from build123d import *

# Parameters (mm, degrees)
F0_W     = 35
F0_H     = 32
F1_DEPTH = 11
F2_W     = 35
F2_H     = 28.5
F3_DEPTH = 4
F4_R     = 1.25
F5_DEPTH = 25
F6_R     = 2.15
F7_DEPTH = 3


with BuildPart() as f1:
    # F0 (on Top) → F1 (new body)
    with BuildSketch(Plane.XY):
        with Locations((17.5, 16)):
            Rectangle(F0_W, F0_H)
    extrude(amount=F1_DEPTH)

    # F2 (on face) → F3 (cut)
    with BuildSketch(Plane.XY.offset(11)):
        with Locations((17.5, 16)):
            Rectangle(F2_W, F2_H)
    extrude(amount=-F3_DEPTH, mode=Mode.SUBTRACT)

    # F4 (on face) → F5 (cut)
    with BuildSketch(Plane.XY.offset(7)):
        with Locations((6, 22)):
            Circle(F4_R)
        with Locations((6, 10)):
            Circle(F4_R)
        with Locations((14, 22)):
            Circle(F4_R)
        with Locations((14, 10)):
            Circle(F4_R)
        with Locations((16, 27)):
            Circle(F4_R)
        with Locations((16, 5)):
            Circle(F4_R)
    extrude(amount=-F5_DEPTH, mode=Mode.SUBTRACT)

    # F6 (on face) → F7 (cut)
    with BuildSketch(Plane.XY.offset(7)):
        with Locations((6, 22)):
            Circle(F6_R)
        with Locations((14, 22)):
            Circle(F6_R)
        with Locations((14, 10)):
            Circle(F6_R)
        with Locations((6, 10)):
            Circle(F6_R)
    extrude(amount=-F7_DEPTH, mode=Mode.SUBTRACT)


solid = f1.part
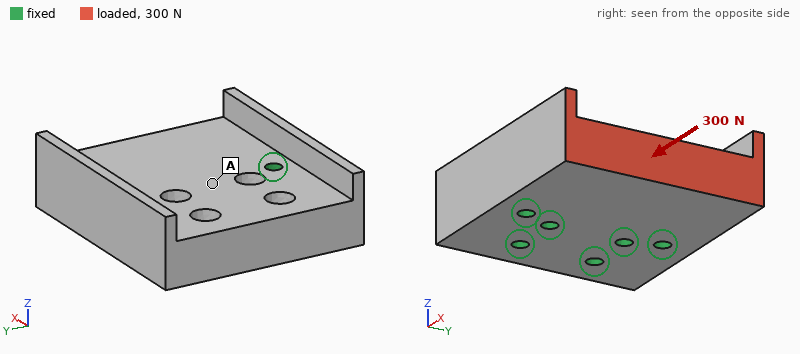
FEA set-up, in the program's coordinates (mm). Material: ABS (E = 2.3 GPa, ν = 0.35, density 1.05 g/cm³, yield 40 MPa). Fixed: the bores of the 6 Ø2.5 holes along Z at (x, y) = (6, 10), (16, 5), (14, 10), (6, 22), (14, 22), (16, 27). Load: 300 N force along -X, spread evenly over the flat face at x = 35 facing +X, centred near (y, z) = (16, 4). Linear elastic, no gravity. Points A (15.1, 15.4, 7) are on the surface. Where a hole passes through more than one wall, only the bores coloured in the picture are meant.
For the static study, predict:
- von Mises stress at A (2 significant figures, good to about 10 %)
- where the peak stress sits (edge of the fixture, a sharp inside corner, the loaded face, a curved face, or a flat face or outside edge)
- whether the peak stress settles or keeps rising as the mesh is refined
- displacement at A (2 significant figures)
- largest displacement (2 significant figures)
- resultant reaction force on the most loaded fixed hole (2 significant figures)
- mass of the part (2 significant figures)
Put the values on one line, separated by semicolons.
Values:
0.74 MPa; edge of the fixture; keeps rising; 3.5 µm; 16 µm; 97 N; 8.4 g
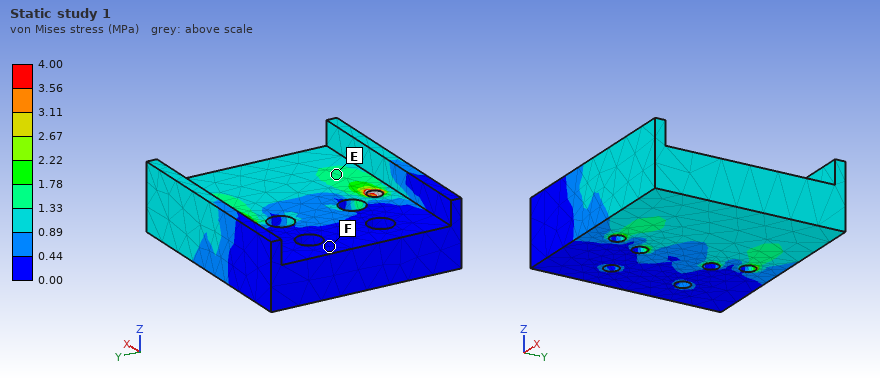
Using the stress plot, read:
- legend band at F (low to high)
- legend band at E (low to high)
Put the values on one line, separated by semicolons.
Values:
0.00 to 0.44 MPa; 1.33 to 1.78 MPa
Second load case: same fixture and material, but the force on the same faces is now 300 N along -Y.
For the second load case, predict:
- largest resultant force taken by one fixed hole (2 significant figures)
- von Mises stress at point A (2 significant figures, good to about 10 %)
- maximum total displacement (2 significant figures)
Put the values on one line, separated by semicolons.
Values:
240 N; 1.1 MPa; 0.12 mm
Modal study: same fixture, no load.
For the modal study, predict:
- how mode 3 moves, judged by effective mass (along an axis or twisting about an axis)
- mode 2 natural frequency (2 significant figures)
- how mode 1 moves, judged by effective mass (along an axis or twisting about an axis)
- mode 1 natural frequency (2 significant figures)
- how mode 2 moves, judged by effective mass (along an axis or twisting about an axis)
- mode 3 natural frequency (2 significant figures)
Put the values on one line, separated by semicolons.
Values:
along Y; 6000 Hz; along Z; 4000 Hz; twisting about X; 8500 Hz
